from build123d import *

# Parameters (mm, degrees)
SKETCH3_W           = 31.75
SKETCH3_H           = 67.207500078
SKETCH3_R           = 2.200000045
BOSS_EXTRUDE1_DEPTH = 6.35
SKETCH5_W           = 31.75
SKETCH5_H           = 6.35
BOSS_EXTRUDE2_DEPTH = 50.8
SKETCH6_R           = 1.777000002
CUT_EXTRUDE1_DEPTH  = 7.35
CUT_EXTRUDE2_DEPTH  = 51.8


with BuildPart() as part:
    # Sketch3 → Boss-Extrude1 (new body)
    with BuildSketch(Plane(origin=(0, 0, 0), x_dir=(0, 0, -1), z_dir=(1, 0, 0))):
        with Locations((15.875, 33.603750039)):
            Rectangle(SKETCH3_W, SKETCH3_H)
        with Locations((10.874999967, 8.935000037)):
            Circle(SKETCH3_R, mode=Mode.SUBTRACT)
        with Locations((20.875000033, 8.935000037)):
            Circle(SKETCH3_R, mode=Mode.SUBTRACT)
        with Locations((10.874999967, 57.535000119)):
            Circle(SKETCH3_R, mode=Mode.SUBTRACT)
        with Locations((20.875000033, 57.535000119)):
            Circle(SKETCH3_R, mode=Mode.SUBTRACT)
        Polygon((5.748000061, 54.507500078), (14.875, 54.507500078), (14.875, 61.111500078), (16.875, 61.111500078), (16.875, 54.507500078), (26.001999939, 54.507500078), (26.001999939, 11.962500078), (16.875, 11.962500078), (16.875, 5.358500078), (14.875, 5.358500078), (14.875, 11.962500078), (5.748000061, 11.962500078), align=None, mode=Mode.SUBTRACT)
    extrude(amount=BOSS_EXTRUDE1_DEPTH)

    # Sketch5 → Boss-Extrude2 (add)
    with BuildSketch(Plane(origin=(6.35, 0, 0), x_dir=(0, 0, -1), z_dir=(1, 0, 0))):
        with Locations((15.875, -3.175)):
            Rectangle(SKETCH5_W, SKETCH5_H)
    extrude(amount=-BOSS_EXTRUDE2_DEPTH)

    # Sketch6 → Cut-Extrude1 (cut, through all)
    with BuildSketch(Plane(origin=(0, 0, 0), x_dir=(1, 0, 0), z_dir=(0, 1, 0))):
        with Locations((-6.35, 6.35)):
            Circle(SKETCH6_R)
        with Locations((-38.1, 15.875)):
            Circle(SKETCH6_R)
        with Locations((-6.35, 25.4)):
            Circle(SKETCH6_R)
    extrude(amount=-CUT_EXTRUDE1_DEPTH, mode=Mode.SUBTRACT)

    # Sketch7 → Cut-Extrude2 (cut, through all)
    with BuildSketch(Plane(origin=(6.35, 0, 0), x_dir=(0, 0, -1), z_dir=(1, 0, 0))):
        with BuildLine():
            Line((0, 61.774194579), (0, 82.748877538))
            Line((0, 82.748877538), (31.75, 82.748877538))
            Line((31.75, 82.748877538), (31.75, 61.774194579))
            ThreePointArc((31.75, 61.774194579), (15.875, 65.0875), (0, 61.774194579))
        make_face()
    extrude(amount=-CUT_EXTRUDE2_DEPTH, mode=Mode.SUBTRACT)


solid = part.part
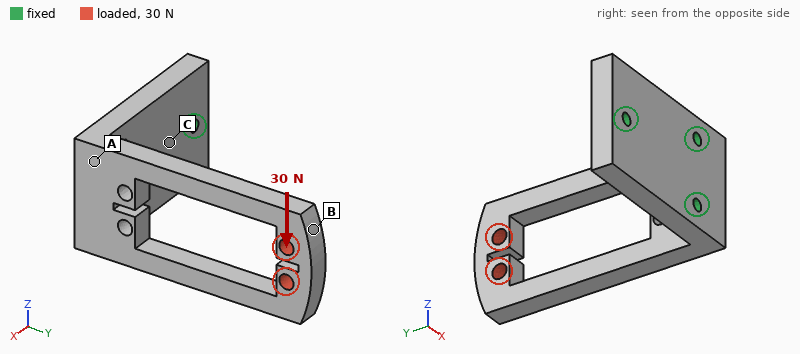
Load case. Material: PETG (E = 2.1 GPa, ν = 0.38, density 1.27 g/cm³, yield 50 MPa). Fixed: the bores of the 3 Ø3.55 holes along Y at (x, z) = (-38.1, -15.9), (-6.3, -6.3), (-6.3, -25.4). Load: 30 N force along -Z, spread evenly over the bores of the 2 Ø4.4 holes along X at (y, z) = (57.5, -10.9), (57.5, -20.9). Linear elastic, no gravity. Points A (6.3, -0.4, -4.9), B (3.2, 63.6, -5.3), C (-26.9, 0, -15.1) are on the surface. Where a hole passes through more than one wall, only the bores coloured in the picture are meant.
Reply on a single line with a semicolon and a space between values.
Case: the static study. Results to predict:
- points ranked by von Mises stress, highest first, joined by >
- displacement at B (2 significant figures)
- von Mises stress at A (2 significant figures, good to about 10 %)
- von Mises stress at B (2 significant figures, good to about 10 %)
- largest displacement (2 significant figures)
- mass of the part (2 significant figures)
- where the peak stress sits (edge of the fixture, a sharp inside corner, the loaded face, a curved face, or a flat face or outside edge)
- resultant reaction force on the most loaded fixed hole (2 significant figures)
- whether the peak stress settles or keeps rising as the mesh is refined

B > A > C; 1.1 mm; 2.2 MPa; 3.3 MPa; 1.1 mm; 22 g; edge of the fixture; 82 N; keeps rising
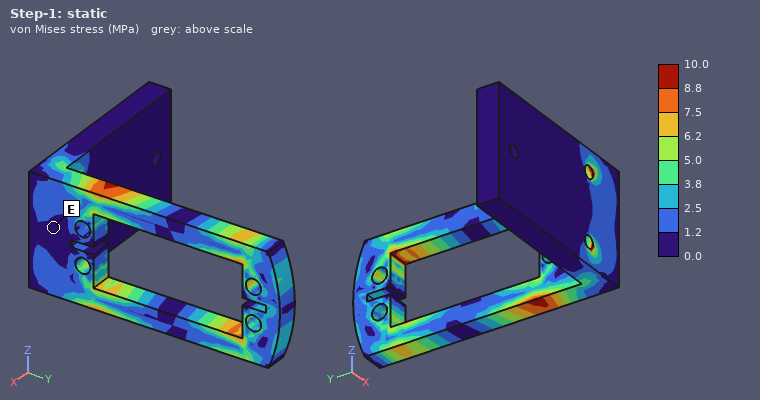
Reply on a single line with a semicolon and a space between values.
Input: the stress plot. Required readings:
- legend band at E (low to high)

0.0 to 1.2 MPa
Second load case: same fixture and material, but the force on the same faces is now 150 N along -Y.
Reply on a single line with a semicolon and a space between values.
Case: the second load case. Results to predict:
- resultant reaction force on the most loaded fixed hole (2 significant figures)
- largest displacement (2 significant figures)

79 N; 0.46 mm
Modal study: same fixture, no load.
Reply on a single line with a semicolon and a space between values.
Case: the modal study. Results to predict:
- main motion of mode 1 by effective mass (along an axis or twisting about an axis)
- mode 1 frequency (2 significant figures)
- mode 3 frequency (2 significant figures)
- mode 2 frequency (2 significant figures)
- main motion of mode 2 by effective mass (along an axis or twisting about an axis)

along X; 240 Hz; 730 Hz; 450 Hz; along Z
